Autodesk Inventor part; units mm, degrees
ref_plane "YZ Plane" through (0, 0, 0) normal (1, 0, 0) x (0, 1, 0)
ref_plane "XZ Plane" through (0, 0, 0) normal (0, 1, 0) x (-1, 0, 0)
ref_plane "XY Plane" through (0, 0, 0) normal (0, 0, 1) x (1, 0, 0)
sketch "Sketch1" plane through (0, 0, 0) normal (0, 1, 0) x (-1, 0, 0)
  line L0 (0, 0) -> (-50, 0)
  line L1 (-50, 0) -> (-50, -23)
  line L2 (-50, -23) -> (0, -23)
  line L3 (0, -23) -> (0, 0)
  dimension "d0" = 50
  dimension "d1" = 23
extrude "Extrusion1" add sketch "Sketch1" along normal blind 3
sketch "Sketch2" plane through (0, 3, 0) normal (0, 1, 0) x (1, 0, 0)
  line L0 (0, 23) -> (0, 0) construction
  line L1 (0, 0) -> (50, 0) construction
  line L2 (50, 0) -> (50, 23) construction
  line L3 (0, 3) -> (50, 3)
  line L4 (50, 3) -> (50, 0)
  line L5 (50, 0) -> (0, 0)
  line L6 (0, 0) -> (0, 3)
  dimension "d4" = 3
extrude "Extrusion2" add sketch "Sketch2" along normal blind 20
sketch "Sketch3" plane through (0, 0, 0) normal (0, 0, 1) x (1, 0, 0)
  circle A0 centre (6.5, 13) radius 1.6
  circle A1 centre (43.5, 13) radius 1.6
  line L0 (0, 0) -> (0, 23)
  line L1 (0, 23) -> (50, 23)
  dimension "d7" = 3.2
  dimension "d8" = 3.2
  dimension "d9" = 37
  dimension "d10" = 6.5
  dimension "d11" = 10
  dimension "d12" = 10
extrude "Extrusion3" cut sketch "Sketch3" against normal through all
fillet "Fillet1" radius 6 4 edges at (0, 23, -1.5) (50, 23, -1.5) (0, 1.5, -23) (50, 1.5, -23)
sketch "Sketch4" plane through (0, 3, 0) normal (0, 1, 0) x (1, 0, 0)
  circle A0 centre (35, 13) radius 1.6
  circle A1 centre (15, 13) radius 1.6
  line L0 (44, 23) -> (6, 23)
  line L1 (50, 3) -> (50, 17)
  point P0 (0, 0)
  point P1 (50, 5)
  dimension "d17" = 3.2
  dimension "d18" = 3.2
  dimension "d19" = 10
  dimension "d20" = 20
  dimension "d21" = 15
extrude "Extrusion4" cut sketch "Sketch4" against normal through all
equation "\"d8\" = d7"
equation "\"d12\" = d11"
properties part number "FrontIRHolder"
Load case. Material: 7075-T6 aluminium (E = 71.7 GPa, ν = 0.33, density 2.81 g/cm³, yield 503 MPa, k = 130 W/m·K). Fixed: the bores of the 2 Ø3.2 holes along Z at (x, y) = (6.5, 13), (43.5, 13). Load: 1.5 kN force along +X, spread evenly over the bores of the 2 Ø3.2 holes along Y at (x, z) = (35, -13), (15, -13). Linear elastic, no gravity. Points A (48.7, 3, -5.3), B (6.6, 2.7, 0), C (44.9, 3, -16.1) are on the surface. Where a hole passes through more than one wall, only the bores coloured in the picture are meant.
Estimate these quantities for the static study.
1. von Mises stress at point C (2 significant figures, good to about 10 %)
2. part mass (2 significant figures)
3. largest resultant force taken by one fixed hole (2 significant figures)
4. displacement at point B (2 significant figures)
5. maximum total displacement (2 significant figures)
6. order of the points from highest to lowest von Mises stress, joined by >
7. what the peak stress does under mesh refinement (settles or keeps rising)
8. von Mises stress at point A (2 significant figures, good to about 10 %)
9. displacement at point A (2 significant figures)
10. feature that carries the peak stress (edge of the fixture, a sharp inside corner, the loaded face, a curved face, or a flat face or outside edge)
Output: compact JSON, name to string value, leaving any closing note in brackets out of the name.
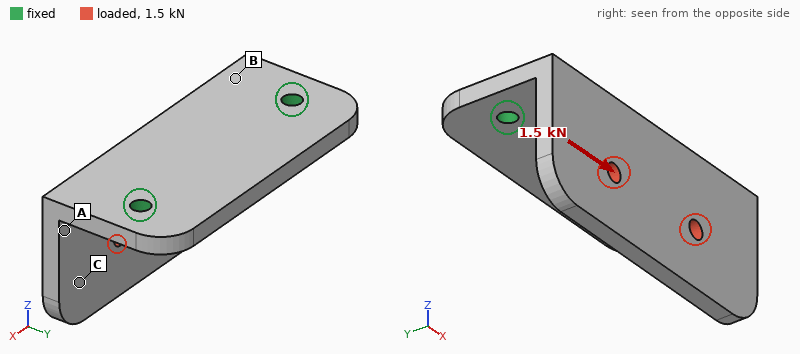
{"von Mises stress at point C": "16 MPa", "part mass": "18 g", "largest resultant force taken by one fixed hole": "980 N", "displacement at point B": "0.045 mm", "maximum total displacement": "0.12 mm", "order of the points from highest to lowest von Mises stress, joined by >": "A > B > C", "what the peak stress does under mesh refinement": "keeps rising", "von Mises stress at point A": "53 MPa", "displacement at point A": "0.064 mm", "feature that carries the peak stress": "edge of the fixture"}
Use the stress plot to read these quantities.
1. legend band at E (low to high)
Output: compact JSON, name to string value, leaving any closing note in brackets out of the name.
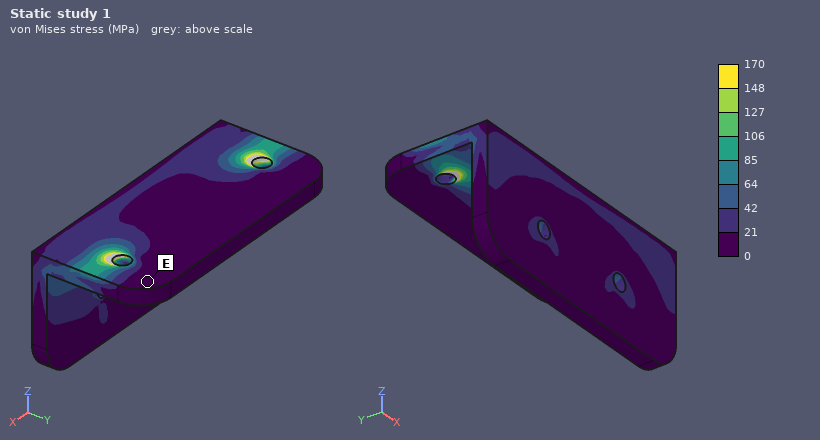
{"legend band at E": "0 to 21 MPa"}
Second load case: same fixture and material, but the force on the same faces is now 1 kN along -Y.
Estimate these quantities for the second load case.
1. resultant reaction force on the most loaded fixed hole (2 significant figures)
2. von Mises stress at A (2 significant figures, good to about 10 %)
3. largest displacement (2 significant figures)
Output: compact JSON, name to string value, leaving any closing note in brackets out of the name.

{"resultant reaction force on the most loaded fixed hole": "520 N", "von Mises stress at A": "65 MPa", "largest displacement": "0.53 mm"}
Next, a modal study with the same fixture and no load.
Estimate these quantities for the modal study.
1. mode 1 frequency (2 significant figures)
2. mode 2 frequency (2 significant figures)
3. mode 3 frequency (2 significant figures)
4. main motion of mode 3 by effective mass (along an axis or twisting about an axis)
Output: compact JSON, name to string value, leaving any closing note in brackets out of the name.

{"mode 1 frequency": "2800 Hz", "mode 2 frequency": "5100 Hz", "mode 3 frequency": "7900 Hz", "main motion of mode 3 by effective mass": "along Z"}
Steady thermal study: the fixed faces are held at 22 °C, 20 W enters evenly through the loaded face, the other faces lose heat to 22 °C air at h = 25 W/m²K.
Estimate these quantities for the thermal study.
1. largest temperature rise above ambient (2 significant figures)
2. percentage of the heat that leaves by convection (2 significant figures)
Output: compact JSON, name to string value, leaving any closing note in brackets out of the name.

{"largest temperature rise above ambient": "31 K", "percentage of the heat that leaves by convection": "8.9 %"}
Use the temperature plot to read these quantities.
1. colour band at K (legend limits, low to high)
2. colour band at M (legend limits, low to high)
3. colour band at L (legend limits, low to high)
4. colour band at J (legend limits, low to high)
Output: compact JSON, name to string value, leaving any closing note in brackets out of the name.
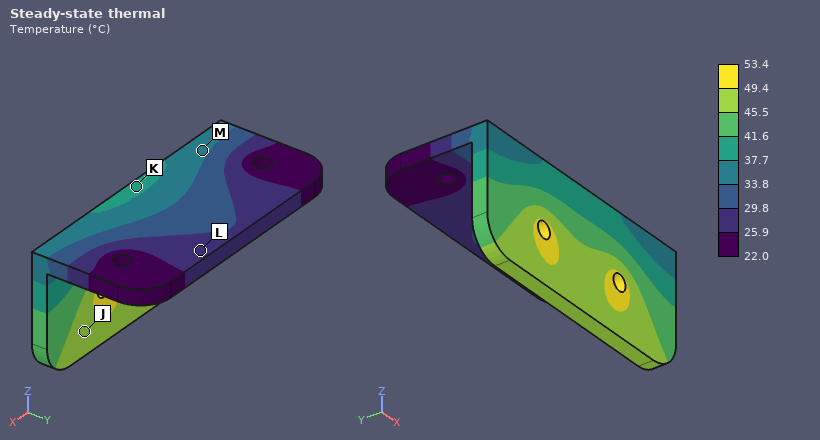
{"colour band at K": "37.7 to 41.6 °C", "colour band at M": "33.8 to 37.7 °C", "colour band at L": "25.9 to 29.8 °C", "colour band at J": "45.5 to 49.4 °C"}
